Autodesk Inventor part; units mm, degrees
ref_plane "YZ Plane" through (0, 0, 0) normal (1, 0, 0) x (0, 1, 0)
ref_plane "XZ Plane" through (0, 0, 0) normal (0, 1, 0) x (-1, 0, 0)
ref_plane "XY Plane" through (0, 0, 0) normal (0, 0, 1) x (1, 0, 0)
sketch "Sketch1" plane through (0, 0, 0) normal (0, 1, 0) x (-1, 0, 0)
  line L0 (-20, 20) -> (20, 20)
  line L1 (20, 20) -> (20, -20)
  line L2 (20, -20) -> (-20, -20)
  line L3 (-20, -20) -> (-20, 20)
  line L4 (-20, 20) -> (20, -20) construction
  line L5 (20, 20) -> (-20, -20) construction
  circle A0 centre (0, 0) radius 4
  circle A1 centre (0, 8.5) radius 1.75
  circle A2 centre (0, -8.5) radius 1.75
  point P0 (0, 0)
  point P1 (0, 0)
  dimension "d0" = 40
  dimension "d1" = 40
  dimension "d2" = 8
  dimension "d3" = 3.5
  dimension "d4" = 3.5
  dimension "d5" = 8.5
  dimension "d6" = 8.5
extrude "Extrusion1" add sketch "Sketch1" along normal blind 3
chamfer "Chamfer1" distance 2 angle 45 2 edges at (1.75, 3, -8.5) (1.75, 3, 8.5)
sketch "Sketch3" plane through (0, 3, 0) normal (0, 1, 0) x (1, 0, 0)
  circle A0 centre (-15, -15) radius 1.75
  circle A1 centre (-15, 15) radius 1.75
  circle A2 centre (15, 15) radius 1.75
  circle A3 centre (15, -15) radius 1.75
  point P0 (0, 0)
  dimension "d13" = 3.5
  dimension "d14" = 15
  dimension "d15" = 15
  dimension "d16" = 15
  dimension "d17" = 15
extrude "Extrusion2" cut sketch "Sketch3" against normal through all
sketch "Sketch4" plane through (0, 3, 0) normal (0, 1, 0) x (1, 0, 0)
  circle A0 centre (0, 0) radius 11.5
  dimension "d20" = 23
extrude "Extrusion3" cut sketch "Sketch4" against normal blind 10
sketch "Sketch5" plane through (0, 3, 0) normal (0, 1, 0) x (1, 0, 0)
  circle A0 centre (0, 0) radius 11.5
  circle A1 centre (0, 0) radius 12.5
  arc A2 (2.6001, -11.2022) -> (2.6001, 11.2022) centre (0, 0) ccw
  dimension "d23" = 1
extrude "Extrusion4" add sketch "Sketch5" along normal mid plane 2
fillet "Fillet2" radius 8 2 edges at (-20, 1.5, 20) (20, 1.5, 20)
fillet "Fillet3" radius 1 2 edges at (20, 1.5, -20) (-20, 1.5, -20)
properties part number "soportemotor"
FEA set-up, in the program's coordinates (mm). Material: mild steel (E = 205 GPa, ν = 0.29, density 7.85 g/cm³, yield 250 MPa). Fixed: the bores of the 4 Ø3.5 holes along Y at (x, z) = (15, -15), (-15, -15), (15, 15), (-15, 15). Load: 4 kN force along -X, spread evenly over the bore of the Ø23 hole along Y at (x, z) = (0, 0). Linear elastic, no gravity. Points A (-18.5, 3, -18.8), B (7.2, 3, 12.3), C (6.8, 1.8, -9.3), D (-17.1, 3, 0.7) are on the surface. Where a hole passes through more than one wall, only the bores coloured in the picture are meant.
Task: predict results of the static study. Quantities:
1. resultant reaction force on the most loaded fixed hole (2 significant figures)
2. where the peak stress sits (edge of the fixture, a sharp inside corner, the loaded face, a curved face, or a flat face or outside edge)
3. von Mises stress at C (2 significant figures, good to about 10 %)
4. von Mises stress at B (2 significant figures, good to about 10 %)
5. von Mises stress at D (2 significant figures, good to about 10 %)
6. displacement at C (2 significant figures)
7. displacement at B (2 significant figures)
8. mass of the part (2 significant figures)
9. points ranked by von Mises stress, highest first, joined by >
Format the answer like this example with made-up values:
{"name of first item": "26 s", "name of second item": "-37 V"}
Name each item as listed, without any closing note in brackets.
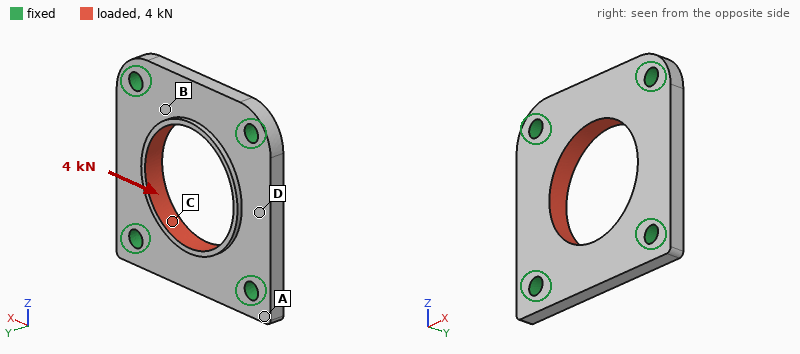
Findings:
{"resultant reaction force on the most loaded fixed hole": "1.0 kN", "where the peak stress sits": "edge of the fixture", "von Mises stress at C": "45 MPa", "von Mises stress at B": "33 MPa", "von Mises stress at D": "20 MPa", "displacement at C": "2.2 µm", "displacement at B": "1.5 µm", "mass of the part": "27 g", "points ranked by von Mises stress, highest first, joined by >": "C > B > D > A"}
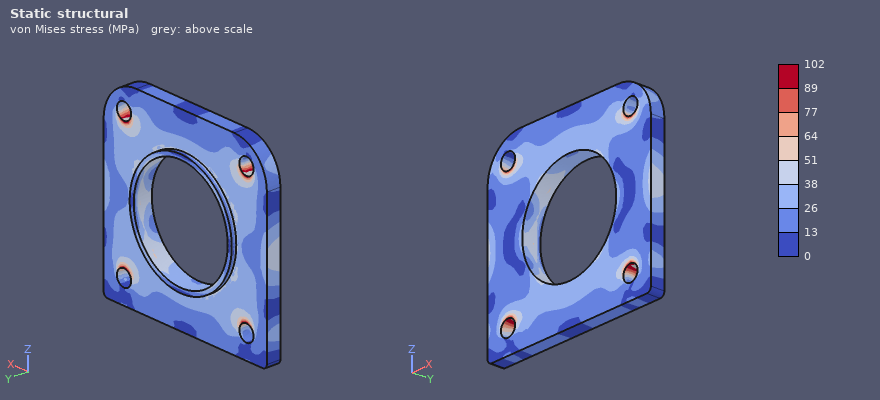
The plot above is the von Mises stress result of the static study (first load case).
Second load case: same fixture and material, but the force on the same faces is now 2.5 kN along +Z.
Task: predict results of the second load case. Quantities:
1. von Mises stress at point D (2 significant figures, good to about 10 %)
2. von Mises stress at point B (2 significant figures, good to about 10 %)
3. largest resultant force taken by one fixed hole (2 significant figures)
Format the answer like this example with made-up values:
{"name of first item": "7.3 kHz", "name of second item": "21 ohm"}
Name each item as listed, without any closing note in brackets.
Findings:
{"von Mises stress at point D": "11 MPa", "von Mises stress at point B": "24 MPa", "largest resultant force taken by one fixed hole": "640 N"}
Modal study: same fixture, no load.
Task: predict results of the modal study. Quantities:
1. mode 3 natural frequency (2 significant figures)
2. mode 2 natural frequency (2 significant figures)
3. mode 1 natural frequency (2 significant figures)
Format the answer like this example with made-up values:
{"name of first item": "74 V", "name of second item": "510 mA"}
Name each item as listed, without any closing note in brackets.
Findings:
{"mode 3 natural frequency": "20 kHz", "mode 2 natural frequency": "19 kHz", "mode 1 natural frequency": "19 kHz"}
